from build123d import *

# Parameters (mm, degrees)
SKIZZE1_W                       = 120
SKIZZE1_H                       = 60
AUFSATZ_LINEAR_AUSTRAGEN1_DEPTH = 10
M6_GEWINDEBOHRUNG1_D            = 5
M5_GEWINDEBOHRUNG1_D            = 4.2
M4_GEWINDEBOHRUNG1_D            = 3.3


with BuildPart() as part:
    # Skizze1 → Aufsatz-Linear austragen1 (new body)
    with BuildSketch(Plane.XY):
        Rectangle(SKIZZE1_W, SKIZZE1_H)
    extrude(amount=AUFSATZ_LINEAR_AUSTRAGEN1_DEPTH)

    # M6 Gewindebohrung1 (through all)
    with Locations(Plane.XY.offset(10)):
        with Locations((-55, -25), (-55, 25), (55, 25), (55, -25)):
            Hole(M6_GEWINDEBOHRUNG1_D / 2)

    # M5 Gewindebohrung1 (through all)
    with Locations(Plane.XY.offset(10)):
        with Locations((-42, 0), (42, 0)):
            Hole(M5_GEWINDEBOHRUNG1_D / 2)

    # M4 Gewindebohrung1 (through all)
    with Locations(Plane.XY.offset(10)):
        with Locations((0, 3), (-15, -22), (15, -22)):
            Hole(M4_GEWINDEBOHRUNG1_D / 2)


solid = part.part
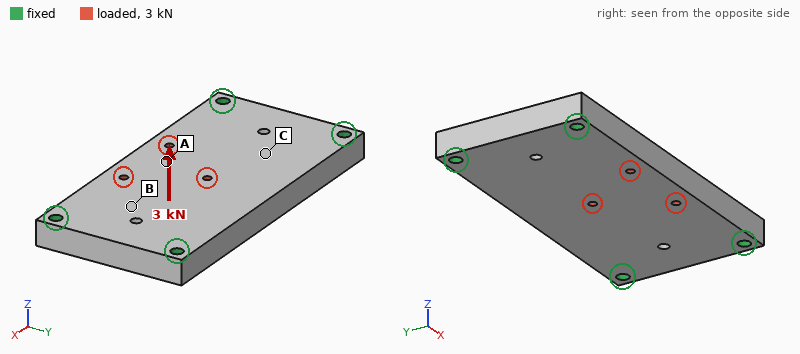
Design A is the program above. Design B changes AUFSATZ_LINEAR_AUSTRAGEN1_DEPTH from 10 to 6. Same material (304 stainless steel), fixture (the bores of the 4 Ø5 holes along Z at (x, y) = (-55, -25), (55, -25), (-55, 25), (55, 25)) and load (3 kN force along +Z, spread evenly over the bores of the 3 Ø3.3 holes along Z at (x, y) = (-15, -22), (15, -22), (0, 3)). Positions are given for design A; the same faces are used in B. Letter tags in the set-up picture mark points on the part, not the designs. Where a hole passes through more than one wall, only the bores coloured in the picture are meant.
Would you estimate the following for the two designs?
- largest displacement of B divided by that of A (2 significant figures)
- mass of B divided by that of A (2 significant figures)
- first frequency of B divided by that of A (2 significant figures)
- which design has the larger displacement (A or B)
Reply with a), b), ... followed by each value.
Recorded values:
a) 4.1
b) 0.60
c) 0.64
d) B
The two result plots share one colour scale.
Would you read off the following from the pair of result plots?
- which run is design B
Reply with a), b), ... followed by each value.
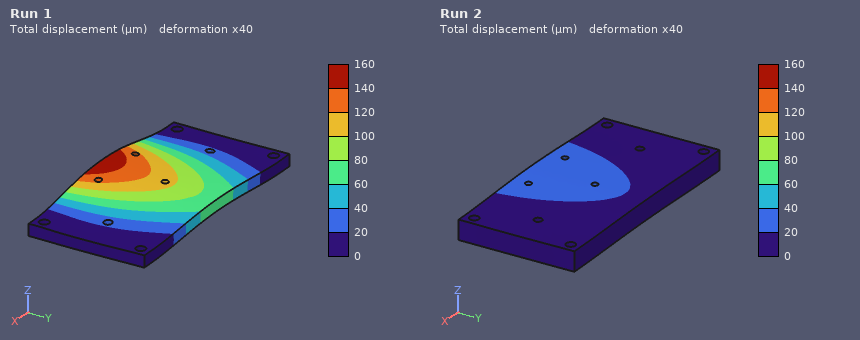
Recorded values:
a) Run 1
